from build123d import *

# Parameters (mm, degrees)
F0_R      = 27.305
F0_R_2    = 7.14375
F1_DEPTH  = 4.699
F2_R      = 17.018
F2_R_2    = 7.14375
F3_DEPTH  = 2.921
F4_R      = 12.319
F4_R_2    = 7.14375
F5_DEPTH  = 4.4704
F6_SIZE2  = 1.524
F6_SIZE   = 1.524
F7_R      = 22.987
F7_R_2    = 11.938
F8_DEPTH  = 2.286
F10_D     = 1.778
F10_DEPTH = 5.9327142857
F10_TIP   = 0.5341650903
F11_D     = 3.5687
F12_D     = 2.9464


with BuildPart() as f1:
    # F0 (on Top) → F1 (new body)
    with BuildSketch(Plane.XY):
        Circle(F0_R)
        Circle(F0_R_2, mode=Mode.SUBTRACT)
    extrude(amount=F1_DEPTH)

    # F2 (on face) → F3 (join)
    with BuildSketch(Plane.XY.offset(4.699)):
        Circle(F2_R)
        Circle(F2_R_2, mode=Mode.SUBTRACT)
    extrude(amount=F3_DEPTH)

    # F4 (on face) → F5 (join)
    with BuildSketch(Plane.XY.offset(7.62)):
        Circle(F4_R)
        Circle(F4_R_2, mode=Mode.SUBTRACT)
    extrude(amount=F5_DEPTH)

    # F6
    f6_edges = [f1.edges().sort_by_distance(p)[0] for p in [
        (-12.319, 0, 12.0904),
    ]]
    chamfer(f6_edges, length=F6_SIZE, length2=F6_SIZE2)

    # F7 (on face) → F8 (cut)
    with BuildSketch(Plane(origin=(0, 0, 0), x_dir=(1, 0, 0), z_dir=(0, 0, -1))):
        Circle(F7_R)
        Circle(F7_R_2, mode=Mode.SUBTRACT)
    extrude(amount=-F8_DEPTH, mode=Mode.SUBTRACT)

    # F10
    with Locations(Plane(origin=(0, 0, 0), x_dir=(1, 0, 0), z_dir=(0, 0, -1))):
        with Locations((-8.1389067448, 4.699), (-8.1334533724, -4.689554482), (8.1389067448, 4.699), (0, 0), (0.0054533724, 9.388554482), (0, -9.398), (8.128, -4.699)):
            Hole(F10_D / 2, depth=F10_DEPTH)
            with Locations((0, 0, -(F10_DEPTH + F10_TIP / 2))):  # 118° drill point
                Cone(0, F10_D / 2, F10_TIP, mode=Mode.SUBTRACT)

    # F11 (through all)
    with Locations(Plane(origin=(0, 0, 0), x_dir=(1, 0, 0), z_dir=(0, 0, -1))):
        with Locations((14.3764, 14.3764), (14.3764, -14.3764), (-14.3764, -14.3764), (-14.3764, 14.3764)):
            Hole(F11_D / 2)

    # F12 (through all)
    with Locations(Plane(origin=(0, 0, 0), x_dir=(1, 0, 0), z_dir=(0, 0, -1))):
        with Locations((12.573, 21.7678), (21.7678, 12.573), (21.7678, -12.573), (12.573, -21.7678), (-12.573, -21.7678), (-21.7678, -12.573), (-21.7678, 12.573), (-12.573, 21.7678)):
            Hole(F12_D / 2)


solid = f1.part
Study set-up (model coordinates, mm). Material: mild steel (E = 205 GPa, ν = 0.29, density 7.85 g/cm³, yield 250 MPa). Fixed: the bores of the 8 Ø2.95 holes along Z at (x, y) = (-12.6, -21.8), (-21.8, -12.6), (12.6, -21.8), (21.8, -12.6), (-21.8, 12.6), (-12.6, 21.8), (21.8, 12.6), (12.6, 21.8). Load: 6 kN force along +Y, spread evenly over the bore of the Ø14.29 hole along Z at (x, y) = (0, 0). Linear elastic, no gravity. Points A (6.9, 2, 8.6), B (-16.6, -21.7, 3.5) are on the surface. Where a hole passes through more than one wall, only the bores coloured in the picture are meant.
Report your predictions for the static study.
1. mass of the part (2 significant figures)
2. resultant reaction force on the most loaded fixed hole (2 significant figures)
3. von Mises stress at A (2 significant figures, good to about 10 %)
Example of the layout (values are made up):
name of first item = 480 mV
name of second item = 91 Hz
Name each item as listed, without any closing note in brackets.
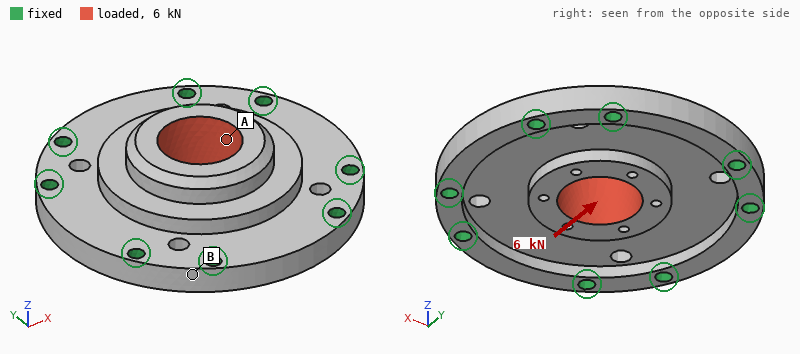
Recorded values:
mass of the part = 83 g
resultant reaction force on the most loaded fixed hole = 1000 N
von Mises stress at A = 24 MPa
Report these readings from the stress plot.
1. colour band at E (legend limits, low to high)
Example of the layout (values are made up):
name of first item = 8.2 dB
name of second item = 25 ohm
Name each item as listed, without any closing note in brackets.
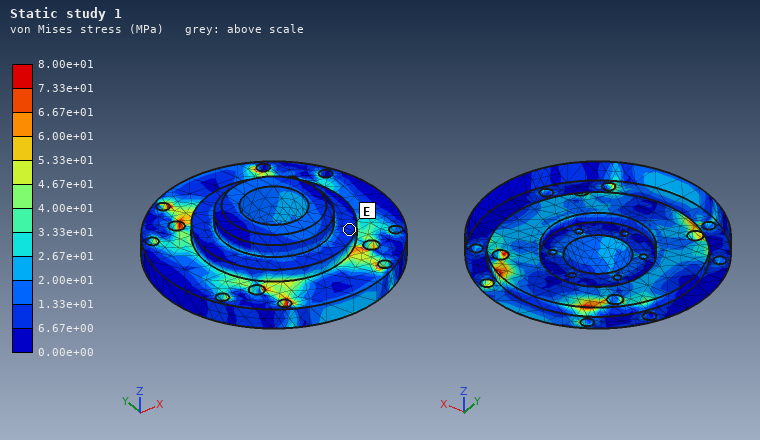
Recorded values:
colour band at E = 6.67e+00 to 1.33e+01 MPa
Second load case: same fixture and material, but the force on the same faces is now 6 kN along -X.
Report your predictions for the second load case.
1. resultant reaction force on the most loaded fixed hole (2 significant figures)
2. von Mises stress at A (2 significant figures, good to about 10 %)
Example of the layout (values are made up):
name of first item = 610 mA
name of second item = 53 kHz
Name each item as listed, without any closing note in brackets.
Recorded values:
resultant reaction force on the most loaded fixed hole = 1.0 kN
von Mises stress at A = 15 MPa
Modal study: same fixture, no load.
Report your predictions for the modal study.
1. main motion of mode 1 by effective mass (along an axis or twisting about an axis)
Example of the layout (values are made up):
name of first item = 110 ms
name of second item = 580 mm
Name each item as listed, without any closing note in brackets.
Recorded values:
main motion of mode 1 by effective mass = along Z
